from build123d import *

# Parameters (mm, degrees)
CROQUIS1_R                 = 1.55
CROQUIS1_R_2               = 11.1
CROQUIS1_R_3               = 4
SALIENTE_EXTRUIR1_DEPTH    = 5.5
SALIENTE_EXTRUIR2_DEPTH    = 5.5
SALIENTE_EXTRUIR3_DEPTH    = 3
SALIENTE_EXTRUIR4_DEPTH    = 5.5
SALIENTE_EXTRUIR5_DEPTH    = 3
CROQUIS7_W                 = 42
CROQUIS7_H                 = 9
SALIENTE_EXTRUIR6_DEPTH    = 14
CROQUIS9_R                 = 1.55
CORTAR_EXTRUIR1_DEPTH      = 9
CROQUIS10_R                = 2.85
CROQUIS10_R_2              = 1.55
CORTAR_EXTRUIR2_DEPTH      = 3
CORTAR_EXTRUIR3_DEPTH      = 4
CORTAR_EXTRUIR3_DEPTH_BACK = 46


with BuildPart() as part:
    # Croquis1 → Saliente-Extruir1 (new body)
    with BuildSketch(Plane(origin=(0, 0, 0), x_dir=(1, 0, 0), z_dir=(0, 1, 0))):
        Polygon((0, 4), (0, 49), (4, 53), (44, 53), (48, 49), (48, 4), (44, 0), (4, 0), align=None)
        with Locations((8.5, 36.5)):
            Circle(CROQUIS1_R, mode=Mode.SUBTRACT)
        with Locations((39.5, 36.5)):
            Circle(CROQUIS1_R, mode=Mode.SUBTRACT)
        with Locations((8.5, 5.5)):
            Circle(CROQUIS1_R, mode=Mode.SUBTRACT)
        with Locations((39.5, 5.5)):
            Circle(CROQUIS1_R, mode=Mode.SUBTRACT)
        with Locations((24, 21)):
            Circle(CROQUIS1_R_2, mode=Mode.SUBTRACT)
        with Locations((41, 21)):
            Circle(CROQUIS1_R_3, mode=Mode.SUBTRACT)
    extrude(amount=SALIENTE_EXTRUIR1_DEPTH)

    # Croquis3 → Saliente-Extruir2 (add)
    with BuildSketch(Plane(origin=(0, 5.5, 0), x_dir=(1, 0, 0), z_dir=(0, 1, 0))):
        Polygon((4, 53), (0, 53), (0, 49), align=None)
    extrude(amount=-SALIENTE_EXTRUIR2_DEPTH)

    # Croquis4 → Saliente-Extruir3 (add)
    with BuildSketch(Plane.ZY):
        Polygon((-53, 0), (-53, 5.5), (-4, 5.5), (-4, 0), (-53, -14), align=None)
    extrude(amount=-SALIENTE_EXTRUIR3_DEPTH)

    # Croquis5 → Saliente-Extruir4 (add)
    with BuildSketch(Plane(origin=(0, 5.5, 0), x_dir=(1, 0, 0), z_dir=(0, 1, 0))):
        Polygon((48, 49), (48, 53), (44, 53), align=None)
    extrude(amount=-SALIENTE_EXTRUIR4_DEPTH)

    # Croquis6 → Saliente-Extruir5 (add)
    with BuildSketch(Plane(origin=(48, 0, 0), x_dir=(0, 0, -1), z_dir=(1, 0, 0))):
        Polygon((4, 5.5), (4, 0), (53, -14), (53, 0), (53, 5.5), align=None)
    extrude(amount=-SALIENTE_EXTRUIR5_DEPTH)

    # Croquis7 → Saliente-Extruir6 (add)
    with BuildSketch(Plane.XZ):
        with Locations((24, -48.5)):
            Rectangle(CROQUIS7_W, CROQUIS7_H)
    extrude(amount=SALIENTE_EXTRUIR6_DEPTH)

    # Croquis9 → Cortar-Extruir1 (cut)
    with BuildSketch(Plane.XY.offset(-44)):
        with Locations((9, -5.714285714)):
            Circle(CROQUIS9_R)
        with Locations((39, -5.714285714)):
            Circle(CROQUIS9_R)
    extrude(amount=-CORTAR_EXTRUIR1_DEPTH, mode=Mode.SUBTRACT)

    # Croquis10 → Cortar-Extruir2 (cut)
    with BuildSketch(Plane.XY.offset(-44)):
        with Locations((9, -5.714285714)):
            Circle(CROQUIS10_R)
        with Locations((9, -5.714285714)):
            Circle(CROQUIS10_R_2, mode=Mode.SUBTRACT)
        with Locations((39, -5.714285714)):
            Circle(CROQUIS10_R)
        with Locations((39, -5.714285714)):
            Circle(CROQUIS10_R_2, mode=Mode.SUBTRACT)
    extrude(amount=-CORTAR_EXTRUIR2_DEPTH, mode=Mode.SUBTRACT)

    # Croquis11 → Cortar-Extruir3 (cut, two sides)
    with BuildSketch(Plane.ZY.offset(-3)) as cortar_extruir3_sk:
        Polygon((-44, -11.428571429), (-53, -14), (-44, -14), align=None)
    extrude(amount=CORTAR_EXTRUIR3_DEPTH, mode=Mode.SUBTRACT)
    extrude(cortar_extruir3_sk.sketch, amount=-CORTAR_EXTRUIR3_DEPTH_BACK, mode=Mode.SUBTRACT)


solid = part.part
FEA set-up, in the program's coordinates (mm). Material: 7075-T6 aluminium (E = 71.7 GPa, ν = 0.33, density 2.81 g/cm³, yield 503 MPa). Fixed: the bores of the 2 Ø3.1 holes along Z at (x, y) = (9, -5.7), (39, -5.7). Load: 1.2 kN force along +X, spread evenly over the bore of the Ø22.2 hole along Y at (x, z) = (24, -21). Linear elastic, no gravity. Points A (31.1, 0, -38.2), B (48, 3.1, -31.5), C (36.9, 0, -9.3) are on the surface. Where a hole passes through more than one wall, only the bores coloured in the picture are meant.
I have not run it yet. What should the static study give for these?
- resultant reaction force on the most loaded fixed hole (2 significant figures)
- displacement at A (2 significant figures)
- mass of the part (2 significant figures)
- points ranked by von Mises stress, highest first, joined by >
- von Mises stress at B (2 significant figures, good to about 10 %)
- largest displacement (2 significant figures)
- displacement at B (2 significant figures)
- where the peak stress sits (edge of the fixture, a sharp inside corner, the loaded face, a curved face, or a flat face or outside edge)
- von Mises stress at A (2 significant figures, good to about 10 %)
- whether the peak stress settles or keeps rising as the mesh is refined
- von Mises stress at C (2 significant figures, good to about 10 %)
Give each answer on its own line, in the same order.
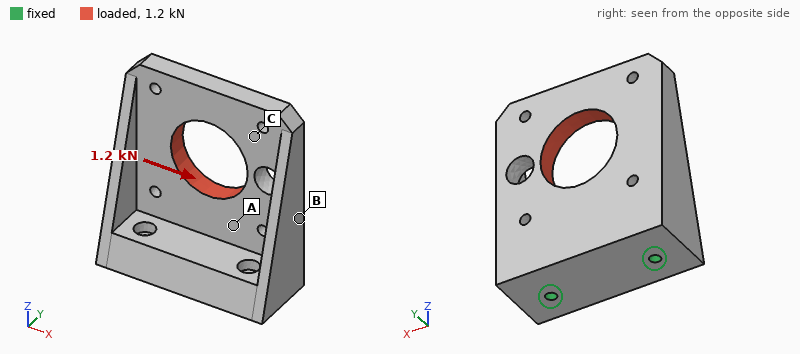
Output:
1.2 kN
8.6 µm
50 g
A > B > C
12 MPa
53 µm
21 µm
edge of the fixture
20 MPa
keeps rising
6.0 MPa
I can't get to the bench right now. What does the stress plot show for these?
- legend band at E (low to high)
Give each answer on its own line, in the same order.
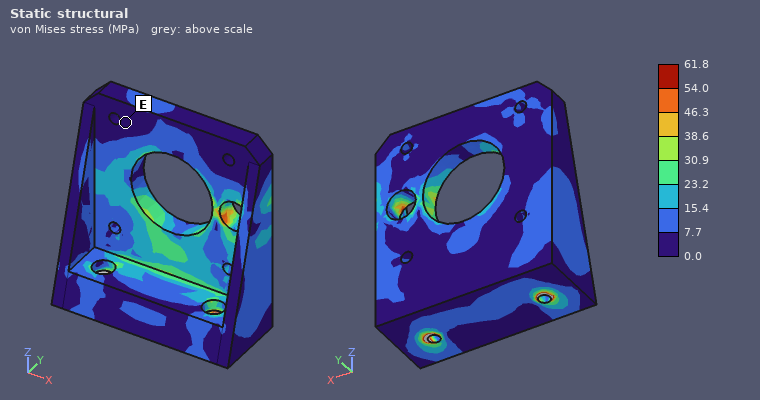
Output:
0.0 to 7.7 MPa
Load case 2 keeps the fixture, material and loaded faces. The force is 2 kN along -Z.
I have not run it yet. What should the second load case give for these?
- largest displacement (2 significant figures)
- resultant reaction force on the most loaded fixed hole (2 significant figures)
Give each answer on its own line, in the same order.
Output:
79 µm
1.0 kN
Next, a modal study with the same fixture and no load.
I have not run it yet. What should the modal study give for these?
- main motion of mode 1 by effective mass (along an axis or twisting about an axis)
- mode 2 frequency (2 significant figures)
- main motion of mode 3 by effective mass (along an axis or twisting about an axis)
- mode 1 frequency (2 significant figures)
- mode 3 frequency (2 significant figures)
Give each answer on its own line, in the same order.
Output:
along Y
4400 Hz
along X
2500 Hz
7600 Hz
